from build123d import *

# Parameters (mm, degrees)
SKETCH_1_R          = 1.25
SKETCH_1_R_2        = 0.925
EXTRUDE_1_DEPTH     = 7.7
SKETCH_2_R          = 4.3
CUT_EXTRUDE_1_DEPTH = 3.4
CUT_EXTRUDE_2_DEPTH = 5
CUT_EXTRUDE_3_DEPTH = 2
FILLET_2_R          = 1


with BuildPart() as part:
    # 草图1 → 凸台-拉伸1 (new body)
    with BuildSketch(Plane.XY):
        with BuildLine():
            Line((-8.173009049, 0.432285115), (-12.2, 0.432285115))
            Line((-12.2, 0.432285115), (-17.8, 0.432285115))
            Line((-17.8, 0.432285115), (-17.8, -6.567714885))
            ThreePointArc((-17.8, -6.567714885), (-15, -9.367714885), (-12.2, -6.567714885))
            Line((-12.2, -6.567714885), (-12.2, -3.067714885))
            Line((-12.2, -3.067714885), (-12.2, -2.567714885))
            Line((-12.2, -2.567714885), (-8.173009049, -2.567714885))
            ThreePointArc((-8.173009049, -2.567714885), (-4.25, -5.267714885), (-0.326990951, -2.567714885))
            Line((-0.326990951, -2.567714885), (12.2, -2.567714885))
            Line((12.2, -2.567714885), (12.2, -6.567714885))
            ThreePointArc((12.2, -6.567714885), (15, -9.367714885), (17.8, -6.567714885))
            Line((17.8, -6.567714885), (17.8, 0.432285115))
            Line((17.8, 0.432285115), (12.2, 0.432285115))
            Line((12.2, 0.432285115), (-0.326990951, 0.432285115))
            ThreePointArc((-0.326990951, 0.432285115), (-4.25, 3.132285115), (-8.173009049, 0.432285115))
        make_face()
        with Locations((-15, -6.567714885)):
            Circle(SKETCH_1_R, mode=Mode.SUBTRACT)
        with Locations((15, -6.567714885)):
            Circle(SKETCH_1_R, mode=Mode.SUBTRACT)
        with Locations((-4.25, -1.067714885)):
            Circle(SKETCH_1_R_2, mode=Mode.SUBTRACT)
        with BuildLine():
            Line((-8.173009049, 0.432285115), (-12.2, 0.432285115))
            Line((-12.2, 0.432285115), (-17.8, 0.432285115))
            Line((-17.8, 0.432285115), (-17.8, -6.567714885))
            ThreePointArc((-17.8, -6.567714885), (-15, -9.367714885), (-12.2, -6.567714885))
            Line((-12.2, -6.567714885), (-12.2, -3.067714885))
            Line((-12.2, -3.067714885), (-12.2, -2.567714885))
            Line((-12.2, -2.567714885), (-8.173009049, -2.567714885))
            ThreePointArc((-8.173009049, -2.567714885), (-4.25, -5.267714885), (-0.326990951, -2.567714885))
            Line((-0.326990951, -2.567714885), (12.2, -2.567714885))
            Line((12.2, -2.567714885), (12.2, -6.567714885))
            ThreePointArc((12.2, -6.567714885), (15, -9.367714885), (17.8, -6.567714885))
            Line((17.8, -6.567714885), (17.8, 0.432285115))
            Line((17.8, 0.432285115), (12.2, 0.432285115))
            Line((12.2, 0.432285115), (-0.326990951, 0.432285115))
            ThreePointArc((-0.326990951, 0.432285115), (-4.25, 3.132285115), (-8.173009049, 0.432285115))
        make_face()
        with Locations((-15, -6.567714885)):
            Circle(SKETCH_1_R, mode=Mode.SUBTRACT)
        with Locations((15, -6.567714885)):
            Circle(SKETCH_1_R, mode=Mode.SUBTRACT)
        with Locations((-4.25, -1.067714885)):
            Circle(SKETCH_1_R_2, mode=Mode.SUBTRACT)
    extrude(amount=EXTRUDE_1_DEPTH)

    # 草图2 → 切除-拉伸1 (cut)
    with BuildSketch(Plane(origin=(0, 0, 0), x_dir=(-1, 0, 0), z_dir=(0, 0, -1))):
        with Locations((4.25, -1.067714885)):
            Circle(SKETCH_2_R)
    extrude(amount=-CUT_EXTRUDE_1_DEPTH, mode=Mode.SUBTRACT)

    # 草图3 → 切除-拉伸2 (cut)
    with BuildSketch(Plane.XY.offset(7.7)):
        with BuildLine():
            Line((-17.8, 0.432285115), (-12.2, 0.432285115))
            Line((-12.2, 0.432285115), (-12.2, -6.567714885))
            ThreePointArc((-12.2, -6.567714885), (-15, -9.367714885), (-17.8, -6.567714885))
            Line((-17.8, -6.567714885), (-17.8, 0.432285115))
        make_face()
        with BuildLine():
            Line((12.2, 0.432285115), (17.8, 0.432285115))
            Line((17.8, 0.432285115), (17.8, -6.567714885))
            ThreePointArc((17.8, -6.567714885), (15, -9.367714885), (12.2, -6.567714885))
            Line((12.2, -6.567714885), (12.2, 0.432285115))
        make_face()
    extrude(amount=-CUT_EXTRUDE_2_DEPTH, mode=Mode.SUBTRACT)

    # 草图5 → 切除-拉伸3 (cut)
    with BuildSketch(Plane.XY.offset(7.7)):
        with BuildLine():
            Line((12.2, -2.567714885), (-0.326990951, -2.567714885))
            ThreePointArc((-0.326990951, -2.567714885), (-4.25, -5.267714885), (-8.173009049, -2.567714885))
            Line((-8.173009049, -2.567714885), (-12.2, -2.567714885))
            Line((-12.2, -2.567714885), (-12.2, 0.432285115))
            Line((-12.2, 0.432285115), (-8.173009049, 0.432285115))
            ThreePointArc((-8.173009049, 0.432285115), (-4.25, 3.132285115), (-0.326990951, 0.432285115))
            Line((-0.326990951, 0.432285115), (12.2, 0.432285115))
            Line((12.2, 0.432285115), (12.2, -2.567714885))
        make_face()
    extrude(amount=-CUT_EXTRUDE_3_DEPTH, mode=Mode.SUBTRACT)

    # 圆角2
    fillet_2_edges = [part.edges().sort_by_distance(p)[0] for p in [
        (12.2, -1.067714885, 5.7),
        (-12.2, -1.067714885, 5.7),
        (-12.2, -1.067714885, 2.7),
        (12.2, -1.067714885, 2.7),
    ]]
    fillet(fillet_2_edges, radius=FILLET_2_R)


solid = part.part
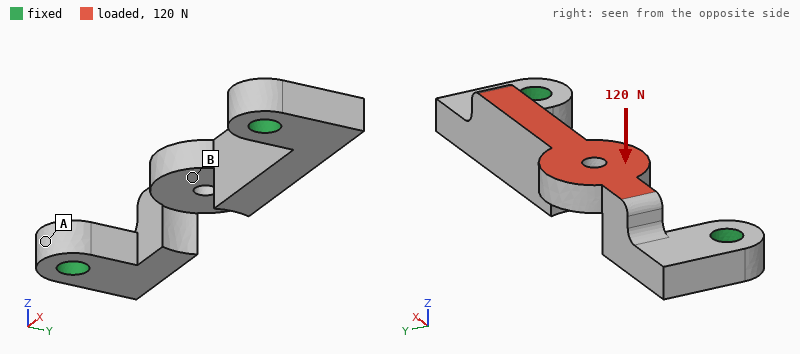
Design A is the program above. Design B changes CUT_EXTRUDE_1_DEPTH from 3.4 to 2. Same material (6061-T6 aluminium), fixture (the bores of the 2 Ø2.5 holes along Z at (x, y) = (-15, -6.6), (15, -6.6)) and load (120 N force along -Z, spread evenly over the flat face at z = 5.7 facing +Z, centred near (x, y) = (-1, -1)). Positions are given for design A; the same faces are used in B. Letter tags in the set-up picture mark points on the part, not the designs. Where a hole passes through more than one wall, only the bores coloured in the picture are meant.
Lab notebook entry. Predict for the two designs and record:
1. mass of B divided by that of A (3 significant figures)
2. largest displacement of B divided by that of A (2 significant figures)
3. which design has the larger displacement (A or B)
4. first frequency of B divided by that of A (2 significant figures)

1.12
0.82
A
0.99
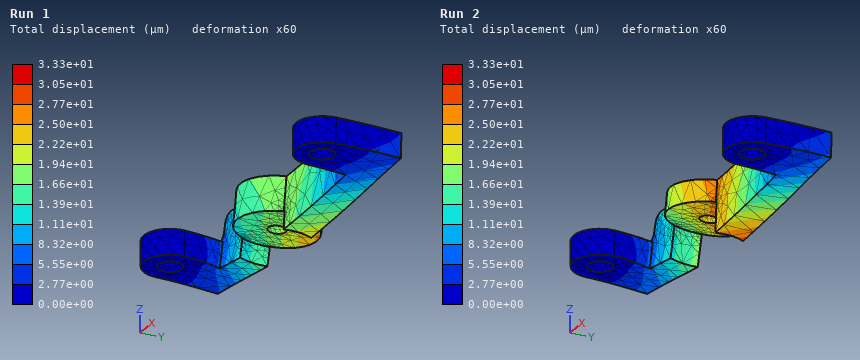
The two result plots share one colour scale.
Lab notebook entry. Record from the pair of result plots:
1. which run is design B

Run 1
